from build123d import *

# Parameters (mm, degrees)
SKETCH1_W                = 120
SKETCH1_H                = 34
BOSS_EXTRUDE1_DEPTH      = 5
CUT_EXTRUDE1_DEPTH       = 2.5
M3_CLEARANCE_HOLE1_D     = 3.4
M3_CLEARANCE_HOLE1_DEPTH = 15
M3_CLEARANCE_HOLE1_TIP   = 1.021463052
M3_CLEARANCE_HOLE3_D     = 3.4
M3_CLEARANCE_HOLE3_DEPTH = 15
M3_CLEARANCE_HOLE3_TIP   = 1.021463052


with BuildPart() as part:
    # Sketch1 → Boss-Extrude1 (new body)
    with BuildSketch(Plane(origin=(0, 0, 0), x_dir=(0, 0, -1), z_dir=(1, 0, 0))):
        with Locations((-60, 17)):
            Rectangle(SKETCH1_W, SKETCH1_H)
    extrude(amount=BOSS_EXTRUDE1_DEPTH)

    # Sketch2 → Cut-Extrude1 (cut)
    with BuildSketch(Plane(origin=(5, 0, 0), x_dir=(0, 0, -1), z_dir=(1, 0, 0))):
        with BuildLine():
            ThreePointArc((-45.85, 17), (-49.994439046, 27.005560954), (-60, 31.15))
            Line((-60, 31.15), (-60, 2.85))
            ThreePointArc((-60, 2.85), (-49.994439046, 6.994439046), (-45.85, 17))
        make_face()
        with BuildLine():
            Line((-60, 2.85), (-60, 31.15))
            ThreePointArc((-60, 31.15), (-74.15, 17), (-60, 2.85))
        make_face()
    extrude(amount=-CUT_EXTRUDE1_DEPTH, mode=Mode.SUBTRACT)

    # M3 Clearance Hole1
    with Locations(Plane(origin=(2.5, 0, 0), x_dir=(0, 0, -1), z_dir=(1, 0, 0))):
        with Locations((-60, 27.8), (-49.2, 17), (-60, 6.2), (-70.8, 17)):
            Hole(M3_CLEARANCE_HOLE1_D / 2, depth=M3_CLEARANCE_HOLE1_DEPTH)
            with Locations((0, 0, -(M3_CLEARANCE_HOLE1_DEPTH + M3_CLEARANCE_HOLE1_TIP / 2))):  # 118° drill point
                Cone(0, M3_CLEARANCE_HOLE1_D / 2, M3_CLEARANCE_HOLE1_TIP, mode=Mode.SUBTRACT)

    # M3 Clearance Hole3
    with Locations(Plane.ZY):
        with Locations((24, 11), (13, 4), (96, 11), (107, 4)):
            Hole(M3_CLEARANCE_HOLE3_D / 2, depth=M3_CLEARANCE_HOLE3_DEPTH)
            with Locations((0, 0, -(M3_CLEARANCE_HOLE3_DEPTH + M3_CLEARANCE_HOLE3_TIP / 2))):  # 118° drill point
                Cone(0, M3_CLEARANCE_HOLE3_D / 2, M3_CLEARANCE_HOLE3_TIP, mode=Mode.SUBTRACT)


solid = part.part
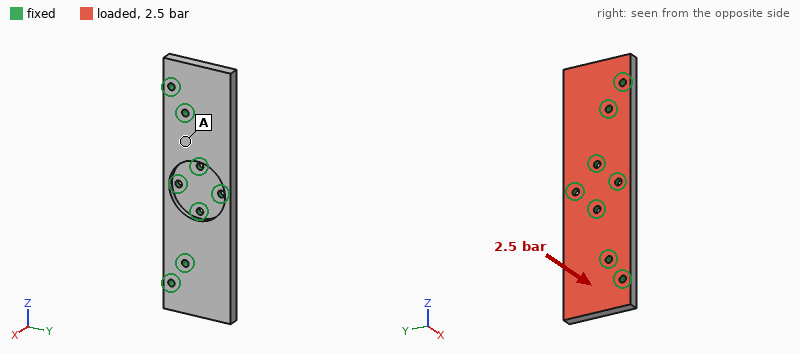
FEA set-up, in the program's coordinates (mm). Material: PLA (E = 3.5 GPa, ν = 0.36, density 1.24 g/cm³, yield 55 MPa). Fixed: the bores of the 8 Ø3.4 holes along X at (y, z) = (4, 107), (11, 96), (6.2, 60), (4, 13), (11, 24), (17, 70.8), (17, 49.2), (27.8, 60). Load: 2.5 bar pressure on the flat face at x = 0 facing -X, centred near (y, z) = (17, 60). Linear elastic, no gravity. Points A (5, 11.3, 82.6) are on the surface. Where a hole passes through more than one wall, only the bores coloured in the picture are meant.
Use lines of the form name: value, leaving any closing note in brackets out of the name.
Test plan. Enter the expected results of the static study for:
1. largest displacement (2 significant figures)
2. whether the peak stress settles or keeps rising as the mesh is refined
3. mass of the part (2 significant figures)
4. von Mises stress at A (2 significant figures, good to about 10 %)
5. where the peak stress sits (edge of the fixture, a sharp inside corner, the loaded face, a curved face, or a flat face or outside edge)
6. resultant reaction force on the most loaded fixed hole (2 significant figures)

largest displacement: 0.50 mm
whether the peak stress settles or keeps rising as the mesh is refined: keeps rising
mass of the part: 23 g
von Mises stress at A: 4.9 MPa
where the peak stress sits: edge of the fixture
resultant reaction force on the most loaded fixed hole: 250 N
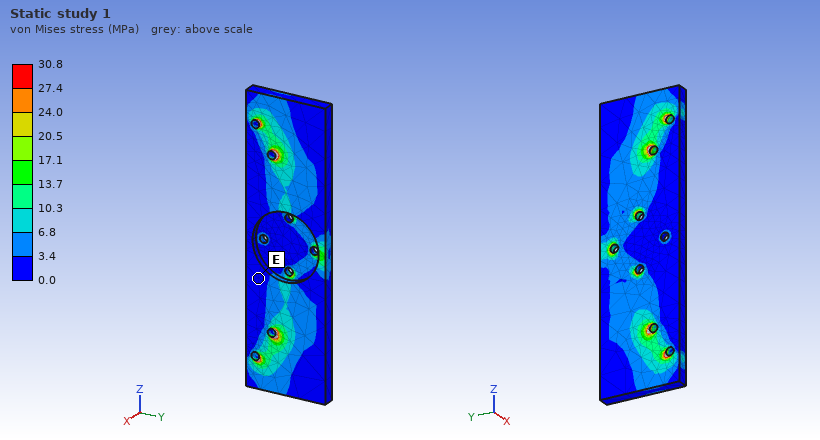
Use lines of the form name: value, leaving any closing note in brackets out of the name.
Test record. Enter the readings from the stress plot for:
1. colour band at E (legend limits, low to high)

colour band at E: 0.0 to 3.4 MPa
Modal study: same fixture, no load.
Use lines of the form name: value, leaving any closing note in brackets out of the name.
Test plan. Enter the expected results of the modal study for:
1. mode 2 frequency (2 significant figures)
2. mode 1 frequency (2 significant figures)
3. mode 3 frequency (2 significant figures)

mode 2 frequency: 2000 Hz
mode 1 frequency: 2000 Hz
mode 3 frequency: 3400 Hz
